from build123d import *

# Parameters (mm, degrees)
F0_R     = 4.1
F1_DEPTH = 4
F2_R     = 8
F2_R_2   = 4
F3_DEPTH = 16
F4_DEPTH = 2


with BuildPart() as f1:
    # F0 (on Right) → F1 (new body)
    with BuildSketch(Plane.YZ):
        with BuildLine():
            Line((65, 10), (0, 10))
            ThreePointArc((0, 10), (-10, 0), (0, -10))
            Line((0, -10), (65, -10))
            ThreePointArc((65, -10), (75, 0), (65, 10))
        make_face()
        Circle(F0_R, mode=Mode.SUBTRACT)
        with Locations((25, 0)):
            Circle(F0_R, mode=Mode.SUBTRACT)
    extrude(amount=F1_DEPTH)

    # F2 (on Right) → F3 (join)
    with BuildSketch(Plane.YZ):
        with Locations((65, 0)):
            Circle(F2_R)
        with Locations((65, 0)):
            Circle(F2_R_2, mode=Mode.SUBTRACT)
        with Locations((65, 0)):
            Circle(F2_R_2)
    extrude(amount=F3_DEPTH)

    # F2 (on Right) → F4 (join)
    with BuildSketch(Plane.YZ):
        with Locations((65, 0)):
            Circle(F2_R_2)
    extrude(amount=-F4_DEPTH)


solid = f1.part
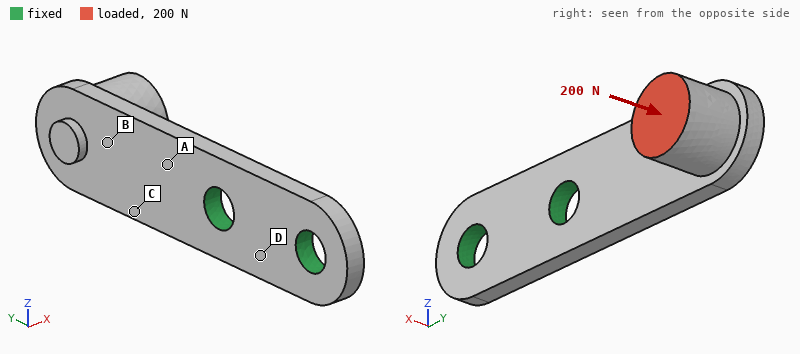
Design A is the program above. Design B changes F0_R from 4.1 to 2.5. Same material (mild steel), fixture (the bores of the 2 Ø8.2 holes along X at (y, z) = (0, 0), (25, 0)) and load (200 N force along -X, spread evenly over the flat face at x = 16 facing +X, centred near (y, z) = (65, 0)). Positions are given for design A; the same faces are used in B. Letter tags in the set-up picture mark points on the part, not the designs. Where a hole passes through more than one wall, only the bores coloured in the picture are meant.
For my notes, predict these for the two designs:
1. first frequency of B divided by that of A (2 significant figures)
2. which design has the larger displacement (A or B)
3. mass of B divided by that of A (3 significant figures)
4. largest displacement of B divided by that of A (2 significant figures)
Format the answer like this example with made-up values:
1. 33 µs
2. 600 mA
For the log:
1. 0.92
2. B
3. 1.03
4. 1.2
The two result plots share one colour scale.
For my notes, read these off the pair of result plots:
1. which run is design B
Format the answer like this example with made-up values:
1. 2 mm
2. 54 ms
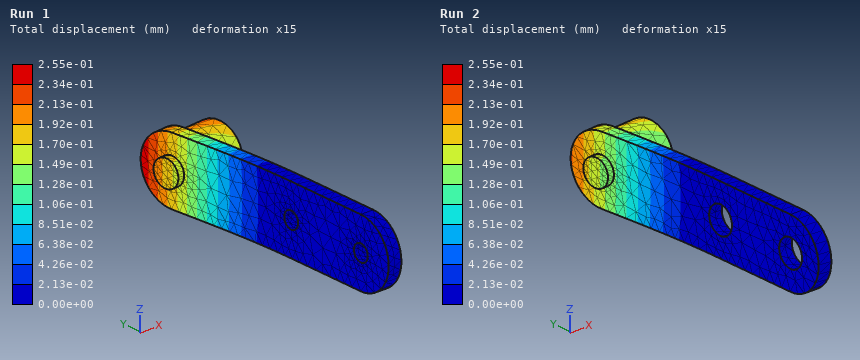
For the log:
1. Run 1
